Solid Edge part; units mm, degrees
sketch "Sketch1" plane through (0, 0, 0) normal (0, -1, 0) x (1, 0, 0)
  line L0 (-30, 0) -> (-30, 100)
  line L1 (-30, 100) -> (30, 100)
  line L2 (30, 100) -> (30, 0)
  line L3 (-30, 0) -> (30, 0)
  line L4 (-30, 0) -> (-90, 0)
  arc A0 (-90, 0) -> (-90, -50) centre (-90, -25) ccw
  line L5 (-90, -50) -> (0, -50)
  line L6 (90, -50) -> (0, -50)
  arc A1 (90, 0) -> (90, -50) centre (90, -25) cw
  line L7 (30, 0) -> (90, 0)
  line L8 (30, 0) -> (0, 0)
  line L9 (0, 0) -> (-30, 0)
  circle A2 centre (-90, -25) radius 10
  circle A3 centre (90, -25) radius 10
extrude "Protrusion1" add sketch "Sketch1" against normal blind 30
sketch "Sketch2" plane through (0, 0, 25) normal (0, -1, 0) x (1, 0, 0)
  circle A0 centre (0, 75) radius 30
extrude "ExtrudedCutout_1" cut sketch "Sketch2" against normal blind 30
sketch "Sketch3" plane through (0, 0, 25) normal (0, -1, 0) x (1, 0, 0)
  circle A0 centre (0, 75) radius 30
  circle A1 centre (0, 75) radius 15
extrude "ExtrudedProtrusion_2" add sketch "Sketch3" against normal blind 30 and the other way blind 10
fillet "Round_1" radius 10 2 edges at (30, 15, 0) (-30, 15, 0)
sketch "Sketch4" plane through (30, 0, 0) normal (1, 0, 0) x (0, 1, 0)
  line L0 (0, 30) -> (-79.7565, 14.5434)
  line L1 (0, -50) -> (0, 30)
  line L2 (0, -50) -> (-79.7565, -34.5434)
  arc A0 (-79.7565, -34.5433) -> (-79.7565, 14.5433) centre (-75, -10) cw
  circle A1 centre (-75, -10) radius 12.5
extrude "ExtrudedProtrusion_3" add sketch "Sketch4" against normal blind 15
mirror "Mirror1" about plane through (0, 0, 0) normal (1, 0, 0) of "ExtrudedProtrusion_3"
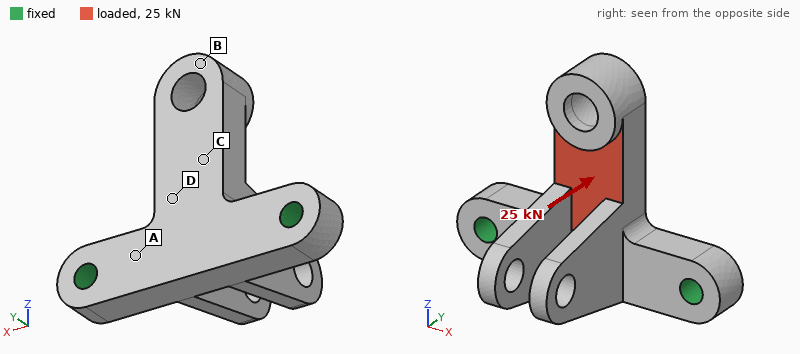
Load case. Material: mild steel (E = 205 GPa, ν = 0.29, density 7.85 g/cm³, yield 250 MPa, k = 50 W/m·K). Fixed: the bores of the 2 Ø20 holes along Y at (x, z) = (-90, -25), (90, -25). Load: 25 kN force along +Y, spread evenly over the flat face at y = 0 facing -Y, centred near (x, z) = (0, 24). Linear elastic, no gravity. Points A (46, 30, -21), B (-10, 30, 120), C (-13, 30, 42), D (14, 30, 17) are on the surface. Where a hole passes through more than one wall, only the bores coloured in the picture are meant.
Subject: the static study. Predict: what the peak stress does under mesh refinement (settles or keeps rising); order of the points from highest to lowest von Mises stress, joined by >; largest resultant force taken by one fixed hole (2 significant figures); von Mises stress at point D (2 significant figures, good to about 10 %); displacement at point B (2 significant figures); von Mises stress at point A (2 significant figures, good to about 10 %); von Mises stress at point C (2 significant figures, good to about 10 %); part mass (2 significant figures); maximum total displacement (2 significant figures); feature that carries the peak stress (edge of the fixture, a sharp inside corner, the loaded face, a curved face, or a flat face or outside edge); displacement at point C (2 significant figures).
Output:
keeps rising
A > D > C > B
13 kN
42 MPa
0.33 mm
88 MPa
24 MPa
5.5 kg
0.36 mm
edge of the fixture
0.16 mm
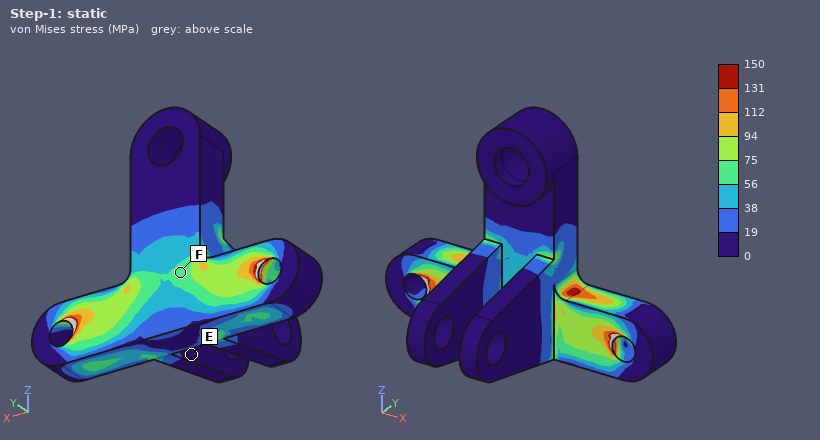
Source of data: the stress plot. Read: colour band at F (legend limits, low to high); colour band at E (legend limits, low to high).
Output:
56 to 75 MPa
0 to 19 MPa
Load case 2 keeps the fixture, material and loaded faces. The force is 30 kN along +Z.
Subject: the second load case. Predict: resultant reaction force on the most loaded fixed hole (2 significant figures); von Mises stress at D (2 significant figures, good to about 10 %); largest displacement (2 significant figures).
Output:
15 kN
17 MPa
0.14 mm
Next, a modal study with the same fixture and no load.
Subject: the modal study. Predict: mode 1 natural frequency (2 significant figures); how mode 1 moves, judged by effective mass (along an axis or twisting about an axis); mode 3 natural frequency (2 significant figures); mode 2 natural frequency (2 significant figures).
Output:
820 Hz
along Y
1500 Hz
1500 Hz
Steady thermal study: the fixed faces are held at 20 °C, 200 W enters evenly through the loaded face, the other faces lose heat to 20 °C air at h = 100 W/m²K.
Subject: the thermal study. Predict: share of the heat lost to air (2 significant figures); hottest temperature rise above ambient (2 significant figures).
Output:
76 %
54 K
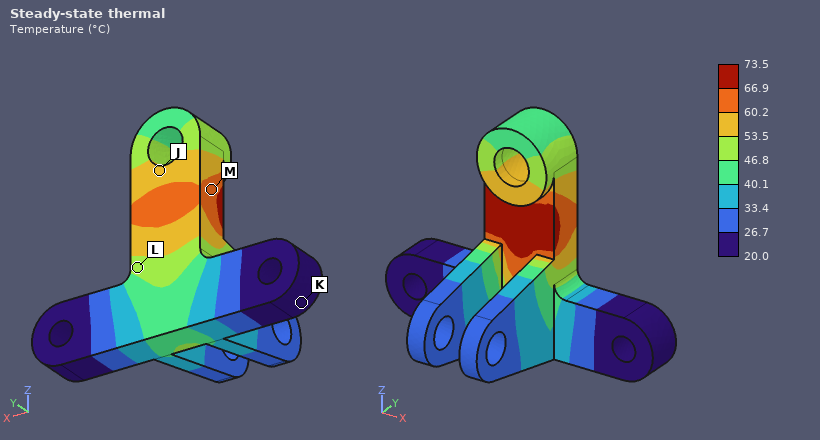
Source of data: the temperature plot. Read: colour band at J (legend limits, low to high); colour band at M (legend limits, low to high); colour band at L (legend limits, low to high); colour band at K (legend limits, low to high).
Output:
53.5 to 60.2 °C
60.2 to 66.9 °C
46.8 to 53.5 °C
20.0 to 26.7 °C
